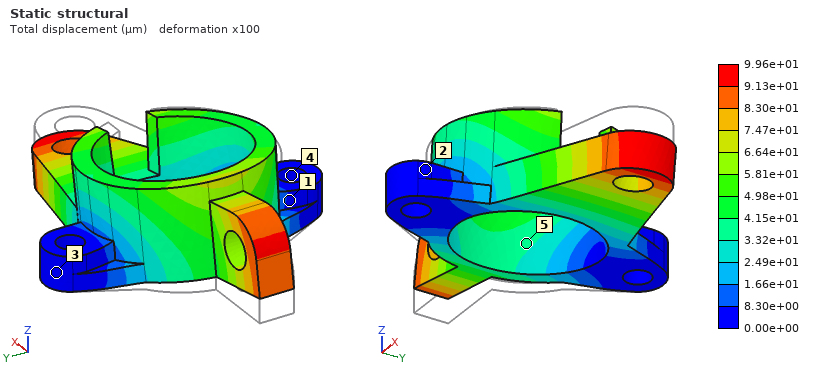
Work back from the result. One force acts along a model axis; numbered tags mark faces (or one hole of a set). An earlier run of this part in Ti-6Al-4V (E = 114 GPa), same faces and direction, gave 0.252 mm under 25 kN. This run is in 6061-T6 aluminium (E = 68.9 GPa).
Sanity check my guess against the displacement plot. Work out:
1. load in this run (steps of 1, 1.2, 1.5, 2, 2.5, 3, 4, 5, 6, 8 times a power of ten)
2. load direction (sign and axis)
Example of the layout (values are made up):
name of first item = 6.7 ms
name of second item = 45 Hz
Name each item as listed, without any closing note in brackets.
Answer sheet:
load in this run = 6 kN
load direction = +X
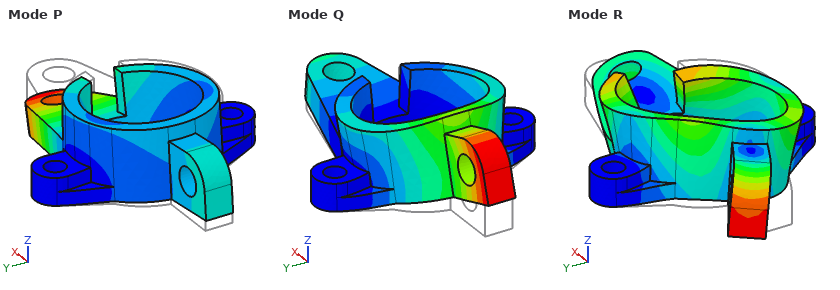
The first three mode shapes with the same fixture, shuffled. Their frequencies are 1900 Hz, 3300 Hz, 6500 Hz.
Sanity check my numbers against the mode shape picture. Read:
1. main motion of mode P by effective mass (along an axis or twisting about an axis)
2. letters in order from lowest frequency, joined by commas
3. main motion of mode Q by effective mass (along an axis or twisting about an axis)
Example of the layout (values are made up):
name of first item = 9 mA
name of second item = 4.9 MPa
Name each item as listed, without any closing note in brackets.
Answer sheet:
main motion of mode P by effective mass = along Z
letters in order from lowest frequency, joined by commas = P, Q, R
main motion of mode Q by effective mass = along Z
